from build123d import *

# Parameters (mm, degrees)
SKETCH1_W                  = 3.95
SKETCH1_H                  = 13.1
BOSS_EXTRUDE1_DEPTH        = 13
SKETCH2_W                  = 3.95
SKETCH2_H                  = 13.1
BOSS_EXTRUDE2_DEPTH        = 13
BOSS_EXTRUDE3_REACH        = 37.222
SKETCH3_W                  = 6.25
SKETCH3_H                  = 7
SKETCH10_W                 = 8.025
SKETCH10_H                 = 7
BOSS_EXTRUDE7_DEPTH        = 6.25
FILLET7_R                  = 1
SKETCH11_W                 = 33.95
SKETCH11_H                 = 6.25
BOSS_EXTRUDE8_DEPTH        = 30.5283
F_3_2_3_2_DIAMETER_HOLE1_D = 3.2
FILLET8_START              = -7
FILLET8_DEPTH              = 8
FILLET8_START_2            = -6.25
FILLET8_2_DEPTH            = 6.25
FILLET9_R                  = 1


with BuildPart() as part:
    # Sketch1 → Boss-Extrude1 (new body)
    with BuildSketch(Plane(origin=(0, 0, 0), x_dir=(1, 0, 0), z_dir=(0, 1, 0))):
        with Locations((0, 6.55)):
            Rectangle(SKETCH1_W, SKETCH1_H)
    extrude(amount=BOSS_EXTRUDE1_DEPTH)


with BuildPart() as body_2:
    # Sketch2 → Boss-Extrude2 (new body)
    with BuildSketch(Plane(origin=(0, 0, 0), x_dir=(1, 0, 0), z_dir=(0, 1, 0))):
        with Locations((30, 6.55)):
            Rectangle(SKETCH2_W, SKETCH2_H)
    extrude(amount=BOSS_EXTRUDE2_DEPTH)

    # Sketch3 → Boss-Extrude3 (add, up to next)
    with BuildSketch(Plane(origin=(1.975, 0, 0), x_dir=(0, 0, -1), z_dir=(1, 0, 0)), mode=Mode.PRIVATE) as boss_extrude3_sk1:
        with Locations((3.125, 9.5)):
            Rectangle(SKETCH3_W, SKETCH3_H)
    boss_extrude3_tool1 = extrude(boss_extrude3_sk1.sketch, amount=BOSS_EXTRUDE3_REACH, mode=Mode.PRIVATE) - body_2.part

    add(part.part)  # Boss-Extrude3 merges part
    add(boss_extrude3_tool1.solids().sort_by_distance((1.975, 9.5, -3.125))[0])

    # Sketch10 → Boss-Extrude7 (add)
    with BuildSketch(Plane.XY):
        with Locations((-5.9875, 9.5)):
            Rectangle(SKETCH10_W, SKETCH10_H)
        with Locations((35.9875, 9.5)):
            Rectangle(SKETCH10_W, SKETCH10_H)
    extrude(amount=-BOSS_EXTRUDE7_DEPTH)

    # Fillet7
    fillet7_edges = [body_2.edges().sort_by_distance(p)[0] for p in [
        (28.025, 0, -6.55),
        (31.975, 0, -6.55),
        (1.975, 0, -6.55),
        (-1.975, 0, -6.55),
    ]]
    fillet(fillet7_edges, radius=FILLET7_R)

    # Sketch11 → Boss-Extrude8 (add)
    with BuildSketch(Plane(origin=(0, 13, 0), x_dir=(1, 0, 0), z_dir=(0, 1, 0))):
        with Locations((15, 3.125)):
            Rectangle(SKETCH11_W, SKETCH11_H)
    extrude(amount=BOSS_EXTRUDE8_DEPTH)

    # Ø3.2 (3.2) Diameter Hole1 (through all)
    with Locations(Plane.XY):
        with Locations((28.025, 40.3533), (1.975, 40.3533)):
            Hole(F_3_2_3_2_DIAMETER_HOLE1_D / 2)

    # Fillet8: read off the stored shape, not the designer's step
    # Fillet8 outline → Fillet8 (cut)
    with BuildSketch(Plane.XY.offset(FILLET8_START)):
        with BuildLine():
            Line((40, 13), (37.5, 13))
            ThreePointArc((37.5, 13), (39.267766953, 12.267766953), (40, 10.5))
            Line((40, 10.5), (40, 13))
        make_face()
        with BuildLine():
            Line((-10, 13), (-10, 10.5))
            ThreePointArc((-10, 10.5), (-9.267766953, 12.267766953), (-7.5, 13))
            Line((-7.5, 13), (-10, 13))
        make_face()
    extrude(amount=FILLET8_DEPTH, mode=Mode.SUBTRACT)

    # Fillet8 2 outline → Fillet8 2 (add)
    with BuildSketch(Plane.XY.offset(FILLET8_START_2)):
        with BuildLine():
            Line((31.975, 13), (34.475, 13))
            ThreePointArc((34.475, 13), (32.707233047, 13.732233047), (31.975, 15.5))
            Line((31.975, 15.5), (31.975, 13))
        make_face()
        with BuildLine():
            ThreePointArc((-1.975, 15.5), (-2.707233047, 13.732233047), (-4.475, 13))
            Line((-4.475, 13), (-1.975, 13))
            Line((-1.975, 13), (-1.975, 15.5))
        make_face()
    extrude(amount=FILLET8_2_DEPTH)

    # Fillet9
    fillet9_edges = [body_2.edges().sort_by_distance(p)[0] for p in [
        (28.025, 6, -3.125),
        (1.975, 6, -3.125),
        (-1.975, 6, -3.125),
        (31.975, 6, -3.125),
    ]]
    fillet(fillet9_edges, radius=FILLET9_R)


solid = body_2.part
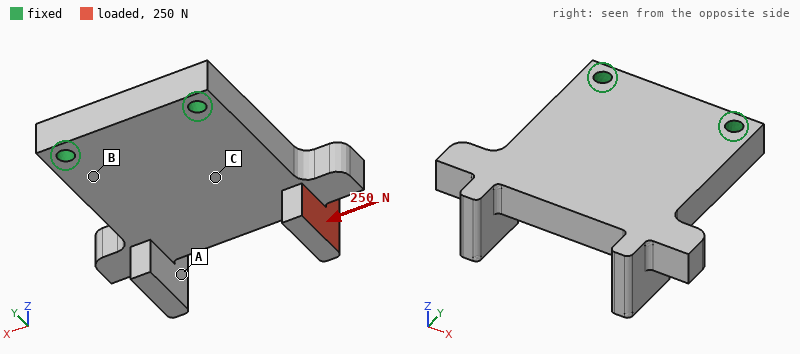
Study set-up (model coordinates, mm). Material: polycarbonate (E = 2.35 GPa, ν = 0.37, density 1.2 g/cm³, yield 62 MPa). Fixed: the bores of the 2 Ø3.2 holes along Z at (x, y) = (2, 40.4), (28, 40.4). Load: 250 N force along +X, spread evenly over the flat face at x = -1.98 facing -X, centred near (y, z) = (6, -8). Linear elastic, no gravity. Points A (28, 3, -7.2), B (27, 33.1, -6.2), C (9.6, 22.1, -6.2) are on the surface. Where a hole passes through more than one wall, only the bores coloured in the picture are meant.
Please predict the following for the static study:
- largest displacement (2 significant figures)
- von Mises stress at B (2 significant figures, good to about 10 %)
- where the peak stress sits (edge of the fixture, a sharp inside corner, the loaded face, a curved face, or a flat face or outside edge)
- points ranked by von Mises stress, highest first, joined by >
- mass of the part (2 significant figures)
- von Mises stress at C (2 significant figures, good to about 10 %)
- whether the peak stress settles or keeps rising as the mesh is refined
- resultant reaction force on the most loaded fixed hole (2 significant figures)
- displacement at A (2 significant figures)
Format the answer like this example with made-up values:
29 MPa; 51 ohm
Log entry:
0.78 mm; 4.6 MPa; a sharp inside corner; C > B > A; 11 g; 8.7 MPa; keeps rising; 340 N; 0.25 mm
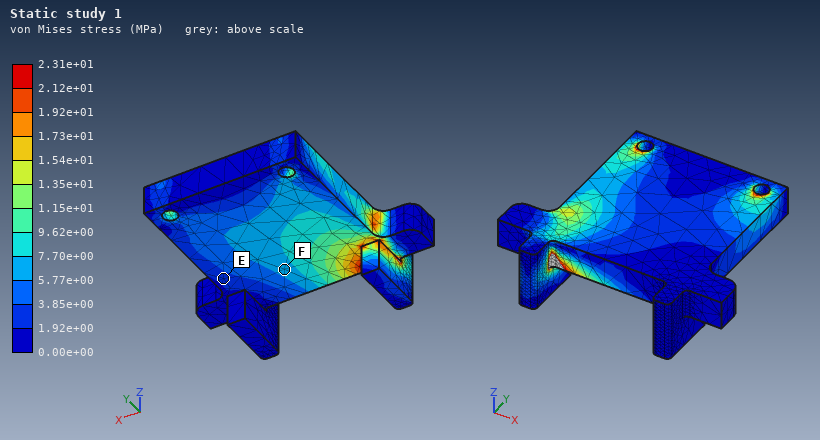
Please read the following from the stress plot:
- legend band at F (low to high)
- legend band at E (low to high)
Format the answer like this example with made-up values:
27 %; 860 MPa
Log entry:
5.77e+00 to 7.70e+00 MPa; 1.92e+00 to 3.85e+00 MPa
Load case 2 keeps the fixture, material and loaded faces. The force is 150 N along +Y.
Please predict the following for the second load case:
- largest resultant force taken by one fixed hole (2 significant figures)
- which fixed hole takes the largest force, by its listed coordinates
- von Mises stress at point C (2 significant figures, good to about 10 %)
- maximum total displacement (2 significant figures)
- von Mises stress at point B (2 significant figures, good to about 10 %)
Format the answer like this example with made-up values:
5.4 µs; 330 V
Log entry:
170 N; (2, 40.4); 4.6 MPa; 0.65 mm; 3.2 MPa
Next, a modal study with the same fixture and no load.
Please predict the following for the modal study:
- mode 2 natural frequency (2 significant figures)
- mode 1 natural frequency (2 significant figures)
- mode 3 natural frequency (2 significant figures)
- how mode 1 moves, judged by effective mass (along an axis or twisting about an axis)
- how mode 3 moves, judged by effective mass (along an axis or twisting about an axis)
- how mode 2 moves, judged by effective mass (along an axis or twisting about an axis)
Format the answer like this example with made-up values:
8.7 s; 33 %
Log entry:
1500 Hz; 760 Hz; 3000 Hz; along Z; along X; twisting about Y
